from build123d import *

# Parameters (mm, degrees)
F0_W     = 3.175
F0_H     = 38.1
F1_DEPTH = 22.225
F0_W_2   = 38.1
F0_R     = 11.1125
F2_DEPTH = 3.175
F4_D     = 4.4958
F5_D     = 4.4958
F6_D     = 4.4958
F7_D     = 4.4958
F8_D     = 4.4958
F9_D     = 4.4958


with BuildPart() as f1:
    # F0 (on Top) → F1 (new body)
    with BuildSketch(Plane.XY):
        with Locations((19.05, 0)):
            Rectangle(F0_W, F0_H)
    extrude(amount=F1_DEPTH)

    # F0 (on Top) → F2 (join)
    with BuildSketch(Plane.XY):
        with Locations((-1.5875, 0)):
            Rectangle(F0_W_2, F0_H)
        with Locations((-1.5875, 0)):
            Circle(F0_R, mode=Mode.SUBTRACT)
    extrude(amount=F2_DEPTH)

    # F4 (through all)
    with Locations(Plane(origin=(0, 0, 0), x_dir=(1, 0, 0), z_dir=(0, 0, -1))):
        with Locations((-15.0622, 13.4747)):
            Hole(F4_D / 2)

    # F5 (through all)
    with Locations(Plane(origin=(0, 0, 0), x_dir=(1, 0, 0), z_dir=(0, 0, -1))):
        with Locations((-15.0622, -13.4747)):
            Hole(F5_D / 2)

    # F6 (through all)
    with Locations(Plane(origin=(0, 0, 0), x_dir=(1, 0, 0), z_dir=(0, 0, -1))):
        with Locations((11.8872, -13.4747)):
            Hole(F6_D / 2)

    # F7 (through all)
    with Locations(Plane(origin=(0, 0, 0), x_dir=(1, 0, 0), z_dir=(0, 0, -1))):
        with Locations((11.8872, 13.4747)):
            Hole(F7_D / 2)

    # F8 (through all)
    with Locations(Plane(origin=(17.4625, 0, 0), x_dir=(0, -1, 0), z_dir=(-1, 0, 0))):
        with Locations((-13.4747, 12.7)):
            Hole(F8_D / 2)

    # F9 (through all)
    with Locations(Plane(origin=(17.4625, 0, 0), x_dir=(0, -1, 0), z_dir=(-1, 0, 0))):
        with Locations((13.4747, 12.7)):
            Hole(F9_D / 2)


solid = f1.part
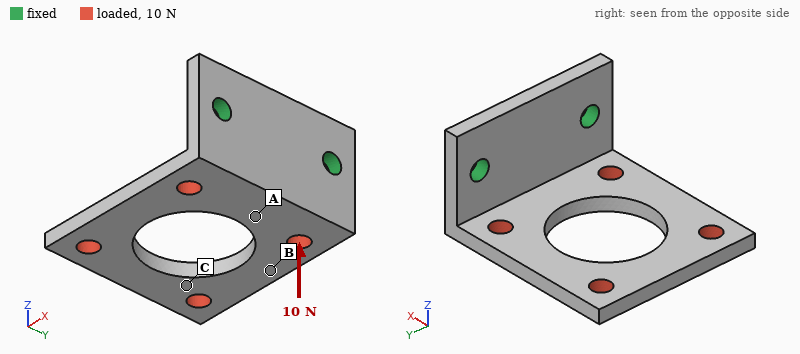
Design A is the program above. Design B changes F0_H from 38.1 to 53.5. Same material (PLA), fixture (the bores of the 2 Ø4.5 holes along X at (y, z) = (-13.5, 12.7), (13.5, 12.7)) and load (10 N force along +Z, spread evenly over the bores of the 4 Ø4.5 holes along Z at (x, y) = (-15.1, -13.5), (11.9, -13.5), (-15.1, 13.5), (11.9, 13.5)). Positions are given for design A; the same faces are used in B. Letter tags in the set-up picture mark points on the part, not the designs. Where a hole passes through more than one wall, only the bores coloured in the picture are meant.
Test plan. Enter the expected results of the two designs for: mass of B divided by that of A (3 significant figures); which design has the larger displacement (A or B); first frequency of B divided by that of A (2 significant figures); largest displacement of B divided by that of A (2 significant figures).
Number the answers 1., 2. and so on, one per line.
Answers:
1. 1.51
2. A
3. 1.00
4. 0.66
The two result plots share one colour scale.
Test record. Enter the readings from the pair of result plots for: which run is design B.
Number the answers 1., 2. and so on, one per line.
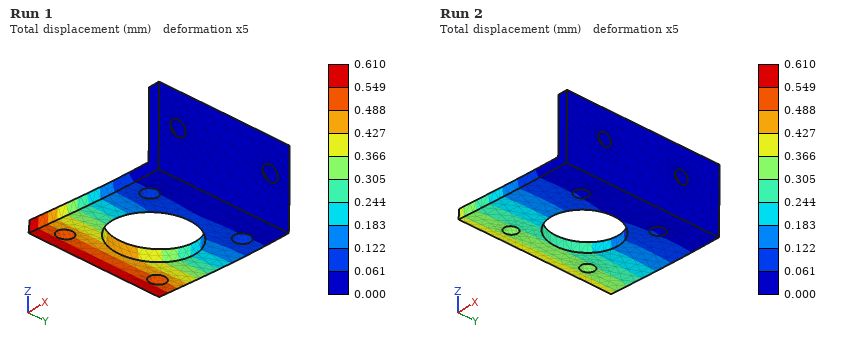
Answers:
1. Run 2
